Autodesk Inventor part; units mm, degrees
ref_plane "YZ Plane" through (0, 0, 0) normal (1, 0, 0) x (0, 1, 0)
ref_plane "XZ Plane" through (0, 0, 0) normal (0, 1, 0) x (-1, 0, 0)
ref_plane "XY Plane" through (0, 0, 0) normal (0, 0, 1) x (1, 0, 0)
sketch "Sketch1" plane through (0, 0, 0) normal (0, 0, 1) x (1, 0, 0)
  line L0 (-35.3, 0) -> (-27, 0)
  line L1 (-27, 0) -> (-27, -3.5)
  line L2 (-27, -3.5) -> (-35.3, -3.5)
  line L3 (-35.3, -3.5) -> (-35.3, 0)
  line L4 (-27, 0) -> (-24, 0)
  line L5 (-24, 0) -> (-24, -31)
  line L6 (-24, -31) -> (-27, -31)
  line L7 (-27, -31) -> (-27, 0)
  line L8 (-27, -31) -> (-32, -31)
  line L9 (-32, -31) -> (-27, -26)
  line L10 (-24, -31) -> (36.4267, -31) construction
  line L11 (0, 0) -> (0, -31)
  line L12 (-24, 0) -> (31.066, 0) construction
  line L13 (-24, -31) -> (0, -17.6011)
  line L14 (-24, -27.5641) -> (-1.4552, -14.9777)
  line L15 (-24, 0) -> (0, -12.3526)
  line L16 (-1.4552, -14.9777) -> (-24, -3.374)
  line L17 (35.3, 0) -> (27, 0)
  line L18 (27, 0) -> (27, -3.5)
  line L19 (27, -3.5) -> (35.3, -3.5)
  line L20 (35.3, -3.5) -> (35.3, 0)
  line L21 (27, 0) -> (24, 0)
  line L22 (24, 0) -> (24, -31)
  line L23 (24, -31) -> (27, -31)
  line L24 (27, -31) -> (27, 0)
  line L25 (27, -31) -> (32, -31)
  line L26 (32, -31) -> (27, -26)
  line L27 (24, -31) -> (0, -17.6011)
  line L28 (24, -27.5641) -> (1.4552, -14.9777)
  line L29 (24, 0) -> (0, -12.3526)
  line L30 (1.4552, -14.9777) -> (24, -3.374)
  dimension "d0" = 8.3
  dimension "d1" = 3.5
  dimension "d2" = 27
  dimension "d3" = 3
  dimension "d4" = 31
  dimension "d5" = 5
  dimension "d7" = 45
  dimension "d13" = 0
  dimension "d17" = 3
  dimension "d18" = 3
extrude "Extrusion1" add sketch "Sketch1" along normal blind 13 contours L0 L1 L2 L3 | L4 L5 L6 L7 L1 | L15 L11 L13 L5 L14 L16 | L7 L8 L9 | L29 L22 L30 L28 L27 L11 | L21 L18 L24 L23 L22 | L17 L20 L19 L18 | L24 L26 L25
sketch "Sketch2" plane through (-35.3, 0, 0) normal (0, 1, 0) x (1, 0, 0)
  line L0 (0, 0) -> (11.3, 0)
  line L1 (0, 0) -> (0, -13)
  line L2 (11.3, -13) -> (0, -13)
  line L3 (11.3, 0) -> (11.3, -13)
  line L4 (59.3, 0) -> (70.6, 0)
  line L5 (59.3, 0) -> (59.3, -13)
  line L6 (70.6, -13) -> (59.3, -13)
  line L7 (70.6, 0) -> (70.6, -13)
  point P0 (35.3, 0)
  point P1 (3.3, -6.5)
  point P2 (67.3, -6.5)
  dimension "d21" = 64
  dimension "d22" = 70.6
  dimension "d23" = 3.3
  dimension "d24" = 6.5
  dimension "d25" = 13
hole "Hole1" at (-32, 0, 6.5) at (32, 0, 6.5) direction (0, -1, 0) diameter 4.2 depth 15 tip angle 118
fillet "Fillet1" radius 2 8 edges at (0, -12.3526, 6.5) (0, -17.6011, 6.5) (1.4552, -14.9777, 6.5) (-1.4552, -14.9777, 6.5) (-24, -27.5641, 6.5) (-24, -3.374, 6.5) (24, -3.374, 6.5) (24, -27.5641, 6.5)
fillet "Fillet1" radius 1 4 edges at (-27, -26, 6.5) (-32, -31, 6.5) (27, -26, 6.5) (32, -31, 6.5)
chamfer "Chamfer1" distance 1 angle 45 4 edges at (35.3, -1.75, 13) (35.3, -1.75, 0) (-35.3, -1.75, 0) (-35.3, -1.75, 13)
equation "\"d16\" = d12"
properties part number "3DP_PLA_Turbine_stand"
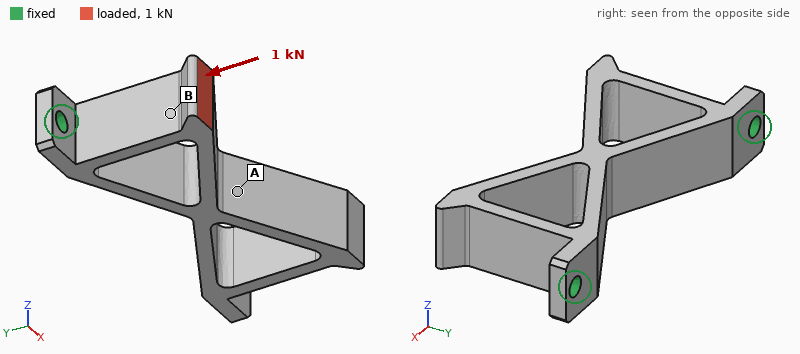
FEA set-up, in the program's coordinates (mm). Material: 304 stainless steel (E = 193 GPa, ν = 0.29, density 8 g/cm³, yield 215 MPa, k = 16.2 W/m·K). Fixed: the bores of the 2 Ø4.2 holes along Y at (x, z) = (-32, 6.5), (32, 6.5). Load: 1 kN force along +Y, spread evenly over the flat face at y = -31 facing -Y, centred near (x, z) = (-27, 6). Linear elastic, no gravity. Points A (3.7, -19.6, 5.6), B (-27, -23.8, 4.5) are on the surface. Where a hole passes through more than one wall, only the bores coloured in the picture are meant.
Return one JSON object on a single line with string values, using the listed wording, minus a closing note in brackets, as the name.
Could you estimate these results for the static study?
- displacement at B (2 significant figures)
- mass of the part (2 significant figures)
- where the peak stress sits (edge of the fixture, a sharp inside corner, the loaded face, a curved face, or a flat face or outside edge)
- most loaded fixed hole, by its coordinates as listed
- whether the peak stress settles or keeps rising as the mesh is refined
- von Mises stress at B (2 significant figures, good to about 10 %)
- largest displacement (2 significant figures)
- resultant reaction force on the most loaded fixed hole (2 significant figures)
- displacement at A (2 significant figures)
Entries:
{"displacement at B": "9.6 µm", "mass of the part": "62 g", "where the peak stress sits": "edge of the fixture", "most loaded fixed hole, by its coordinates as listed": "(-32, 6.5)", "whether the peak stress settles or keeps rising as the mesh is refined": "keeps rising", "von Mises stress at B": "45 MPa", "largest displacement": "15 µm", "resultant reaction force on the most loaded fixed hole": "990 N", "displacement at A": "3.7 µm"}
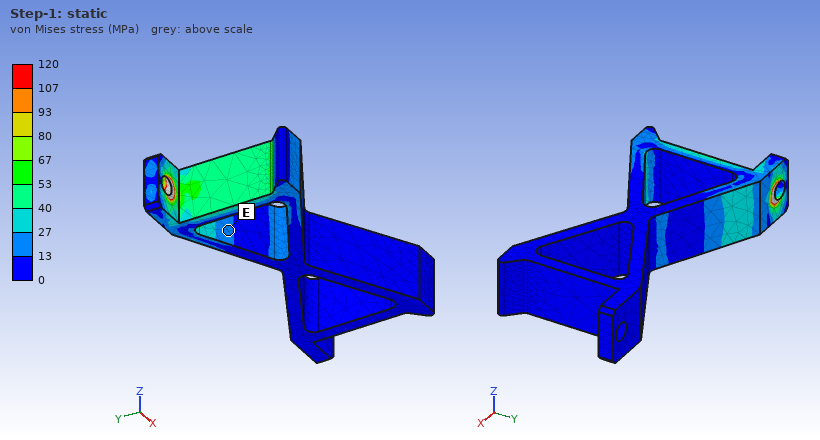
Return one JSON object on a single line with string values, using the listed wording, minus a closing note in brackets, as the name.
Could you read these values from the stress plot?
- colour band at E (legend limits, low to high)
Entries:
{"colour band at E": "13 to 27 MPa"}
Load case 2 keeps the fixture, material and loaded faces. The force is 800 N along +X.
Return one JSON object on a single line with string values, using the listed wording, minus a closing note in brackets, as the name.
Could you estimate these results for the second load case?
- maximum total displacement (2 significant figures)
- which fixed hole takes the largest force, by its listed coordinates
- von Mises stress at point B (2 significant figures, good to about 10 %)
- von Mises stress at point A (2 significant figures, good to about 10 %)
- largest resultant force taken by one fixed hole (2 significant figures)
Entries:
{"maximum total displacement": "17 µm", "which fixed hole takes the largest force, by its listed coordinates": "(32, 6.5)", "von Mises stress at point B": "21 MPa", "von Mises stress at point A": "24 MPa", "largest resultant force taken by one fixed hole": "950 N"}
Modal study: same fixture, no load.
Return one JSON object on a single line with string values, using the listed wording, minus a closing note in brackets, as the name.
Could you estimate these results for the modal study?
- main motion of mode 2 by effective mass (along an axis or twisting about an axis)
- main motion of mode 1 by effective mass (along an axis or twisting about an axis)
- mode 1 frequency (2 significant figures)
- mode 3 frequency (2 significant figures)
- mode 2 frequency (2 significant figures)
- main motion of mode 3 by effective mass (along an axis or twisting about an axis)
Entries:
{"main motion of mode 2 by effective mass": "twisting about Y", "main motion of mode 1 by effective mass": "along Z", "mode 1 frequency": "2800 Hz", "mode 3 frequency": "7700 Hz", "mode 2 frequency": "6000 Hz", "main motion of mode 3 by effective mass": "along Y"}
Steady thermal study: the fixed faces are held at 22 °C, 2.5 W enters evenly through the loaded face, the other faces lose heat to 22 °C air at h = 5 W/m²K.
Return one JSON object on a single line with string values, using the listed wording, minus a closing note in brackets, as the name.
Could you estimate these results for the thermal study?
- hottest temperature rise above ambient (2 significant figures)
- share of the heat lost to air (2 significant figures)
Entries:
{"hottest temperature rise above ambient": "68 K", "share of the heat lost to air": "22 %"}
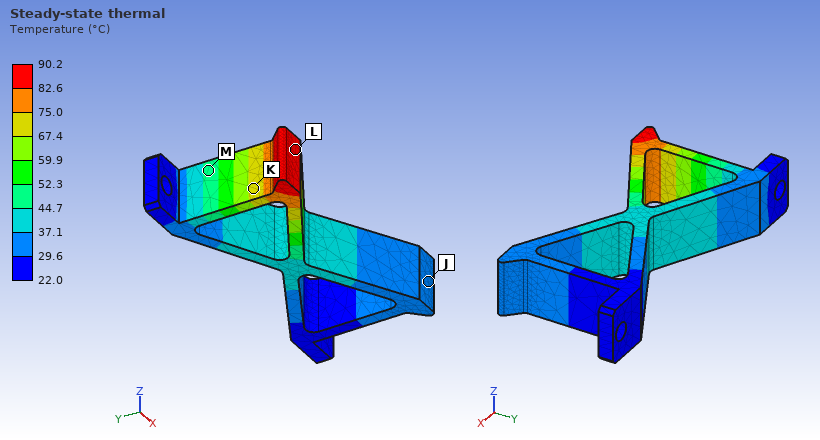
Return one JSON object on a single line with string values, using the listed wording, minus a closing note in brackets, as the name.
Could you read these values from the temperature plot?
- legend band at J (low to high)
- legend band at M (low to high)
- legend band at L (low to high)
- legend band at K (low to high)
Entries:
{"legend band at J": "29.6 to 37.1 °C", "legend band at M": "44.7 to 52.3 °C", "legend band at L": "82.6 to 90.2 °C", "legend band at K": "67.4 to 75.0 °C"}
